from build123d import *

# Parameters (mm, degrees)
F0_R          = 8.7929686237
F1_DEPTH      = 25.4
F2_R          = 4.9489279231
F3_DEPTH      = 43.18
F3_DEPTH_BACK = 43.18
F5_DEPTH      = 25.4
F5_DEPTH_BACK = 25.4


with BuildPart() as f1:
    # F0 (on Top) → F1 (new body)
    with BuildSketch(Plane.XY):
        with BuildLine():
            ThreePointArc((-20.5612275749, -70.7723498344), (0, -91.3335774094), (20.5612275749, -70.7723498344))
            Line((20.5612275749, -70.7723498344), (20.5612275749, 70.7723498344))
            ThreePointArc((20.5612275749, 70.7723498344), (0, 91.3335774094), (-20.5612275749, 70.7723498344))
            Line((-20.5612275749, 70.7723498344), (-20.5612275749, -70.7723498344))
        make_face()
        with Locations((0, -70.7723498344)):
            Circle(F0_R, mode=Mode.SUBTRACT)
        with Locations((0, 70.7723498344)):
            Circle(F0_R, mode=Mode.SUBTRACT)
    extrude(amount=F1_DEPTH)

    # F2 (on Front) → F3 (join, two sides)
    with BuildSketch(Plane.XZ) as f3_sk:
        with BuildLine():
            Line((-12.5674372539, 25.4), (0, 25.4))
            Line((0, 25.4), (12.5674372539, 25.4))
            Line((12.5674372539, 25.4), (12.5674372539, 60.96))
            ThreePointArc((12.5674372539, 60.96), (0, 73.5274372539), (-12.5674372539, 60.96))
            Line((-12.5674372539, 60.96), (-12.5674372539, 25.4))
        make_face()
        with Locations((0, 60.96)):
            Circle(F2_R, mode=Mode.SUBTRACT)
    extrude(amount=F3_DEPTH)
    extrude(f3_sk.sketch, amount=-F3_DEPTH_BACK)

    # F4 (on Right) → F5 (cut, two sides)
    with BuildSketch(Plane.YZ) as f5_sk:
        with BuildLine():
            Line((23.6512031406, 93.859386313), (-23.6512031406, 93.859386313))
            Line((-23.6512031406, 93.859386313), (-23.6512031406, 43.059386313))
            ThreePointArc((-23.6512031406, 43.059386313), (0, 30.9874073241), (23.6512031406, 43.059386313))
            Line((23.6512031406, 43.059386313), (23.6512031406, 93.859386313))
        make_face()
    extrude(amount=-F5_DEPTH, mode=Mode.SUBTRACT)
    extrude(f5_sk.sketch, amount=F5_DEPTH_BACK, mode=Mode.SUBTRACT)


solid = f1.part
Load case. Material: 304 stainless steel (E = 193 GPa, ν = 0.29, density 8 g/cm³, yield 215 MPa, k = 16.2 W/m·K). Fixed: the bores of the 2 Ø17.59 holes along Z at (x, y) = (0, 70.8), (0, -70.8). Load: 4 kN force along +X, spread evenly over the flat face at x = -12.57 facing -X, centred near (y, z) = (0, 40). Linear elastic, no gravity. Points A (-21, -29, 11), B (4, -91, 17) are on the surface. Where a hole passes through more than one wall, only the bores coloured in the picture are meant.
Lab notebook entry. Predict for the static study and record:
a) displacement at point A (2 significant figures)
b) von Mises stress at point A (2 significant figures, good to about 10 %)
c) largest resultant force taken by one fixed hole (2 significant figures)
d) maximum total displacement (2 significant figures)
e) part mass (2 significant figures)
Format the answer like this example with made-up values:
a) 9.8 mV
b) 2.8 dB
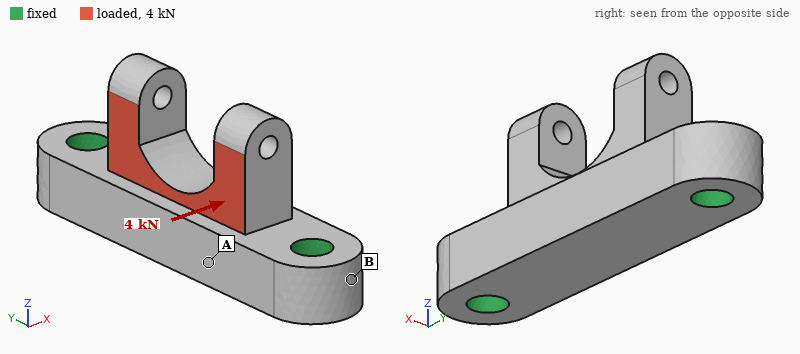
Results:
a) 3.6 µm
b) 5.9 MPa
c) 2.0 kN
d) 15 µm
e) 1.8 kg
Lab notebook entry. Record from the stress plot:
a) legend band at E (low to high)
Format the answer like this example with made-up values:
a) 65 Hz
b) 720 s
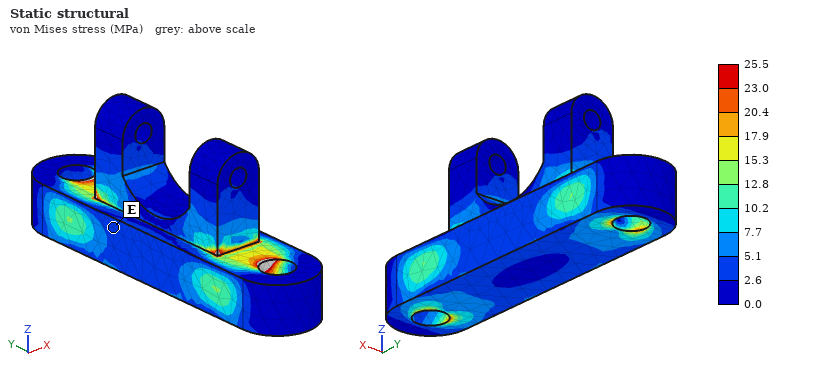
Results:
a) 2.6 to 5.1 MPa
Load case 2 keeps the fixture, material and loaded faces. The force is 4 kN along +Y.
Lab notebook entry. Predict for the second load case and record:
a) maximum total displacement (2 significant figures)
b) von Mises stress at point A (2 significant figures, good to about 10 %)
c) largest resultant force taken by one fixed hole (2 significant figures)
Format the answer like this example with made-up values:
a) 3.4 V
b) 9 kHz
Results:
a) 5.2 µm
b) 1.7 MPa
c) 2.3 kN
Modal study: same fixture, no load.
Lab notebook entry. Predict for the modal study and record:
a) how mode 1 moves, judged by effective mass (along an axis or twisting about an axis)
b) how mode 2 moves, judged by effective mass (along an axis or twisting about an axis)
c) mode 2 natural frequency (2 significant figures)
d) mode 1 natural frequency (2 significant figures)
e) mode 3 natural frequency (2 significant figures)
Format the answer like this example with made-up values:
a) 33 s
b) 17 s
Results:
a) along X
b) along Z
c) 5200 Hz
d) 4200 Hz
e) 6300 Hz
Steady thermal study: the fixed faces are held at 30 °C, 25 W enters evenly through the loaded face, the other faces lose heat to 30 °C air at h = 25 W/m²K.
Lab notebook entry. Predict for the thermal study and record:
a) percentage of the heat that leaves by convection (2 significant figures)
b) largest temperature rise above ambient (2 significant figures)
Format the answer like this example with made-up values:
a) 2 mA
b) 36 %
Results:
a) 41 %
b) 36 K
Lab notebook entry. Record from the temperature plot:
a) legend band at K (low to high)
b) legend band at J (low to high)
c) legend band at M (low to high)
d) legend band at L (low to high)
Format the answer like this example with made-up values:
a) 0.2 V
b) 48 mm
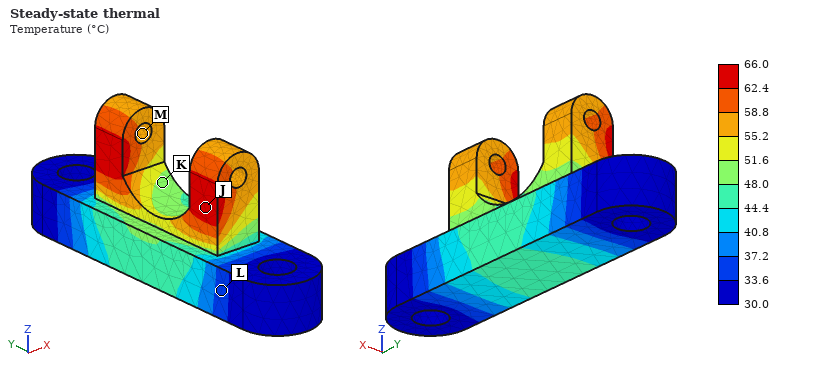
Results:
a) 48.0 to 51.6 °C
b) 62.4 to 66.0 °C
c) 55.2 to 58.8 °C
d) 33.6 to 37.2 °C
